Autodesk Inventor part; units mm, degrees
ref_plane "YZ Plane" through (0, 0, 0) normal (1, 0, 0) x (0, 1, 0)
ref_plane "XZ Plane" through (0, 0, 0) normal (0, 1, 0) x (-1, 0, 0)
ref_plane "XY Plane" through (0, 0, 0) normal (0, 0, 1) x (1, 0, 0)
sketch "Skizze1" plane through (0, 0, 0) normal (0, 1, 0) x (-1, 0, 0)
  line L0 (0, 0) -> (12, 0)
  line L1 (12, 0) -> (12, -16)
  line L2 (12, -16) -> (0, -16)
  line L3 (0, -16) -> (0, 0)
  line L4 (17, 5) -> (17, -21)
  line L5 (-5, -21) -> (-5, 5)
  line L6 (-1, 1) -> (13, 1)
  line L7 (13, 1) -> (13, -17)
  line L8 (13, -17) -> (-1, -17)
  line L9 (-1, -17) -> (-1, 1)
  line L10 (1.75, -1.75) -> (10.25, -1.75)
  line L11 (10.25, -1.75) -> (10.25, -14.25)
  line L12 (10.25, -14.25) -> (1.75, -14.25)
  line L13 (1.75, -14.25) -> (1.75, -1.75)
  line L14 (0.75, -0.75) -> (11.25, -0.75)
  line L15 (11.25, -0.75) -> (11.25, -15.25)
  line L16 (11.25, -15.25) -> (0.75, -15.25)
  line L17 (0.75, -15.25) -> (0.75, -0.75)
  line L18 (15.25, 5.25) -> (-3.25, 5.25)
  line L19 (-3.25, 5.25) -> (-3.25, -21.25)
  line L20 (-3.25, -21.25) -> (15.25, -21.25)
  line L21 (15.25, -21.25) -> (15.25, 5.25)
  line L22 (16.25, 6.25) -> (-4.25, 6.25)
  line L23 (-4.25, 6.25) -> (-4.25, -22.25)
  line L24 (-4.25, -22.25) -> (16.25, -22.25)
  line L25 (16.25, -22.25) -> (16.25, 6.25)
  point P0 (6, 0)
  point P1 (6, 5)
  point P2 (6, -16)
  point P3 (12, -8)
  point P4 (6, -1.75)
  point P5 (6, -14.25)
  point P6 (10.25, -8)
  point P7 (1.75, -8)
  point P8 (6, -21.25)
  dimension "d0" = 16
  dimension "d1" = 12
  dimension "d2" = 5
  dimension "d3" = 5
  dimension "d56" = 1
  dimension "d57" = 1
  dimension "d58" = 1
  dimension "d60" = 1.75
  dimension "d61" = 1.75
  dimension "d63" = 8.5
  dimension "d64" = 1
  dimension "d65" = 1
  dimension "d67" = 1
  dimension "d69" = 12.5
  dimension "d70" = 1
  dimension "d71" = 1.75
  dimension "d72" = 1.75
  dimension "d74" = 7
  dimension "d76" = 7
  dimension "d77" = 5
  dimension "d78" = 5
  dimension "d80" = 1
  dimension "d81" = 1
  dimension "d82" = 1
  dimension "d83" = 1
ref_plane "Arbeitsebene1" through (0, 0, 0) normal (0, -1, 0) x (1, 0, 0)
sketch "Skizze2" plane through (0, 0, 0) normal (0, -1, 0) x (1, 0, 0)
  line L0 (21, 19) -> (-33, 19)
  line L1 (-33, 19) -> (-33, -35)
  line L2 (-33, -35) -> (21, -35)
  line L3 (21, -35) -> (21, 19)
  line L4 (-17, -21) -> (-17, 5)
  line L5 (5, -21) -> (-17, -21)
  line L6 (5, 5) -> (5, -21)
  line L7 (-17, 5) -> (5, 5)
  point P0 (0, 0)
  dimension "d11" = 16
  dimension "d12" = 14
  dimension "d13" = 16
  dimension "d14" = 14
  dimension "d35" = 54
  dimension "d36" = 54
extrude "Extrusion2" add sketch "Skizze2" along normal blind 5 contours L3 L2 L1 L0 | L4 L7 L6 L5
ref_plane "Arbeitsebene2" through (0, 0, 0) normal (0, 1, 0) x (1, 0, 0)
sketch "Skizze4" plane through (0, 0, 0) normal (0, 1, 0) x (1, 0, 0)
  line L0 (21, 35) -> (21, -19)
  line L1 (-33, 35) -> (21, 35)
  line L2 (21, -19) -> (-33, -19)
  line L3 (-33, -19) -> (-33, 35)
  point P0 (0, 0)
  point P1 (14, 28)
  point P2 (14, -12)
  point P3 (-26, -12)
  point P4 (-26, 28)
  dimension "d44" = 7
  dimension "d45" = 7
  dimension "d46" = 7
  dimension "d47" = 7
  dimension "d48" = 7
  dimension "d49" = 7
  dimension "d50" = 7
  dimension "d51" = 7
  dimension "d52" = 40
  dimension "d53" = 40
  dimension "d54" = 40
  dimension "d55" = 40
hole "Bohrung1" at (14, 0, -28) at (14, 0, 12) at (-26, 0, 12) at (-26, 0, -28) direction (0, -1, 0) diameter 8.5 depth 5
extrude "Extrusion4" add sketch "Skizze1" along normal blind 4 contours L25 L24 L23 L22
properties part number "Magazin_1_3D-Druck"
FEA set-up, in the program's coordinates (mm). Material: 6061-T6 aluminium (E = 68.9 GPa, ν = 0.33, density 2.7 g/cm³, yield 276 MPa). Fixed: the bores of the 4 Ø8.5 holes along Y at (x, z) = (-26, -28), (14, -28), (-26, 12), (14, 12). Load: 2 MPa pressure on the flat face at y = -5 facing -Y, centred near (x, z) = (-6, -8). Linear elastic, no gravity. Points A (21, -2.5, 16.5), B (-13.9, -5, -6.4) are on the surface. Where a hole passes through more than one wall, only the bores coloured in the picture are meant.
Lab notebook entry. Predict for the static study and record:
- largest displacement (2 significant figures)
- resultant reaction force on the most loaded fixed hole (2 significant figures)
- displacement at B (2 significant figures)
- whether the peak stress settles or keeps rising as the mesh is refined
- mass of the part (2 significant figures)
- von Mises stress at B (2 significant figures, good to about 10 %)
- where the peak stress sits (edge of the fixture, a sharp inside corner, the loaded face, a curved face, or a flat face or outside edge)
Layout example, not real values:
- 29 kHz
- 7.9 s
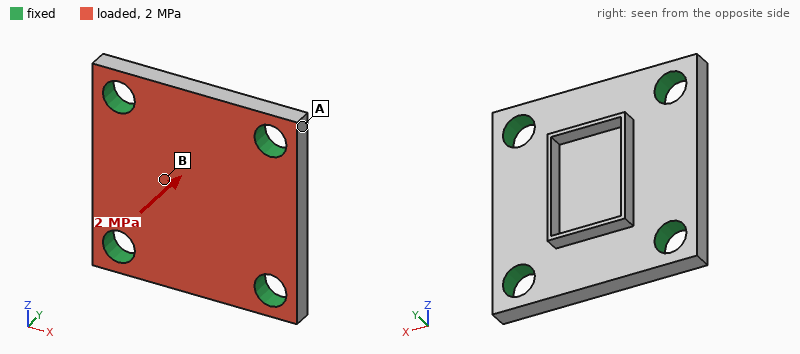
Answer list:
- 27 µm
- 1.3 kN
- 23 µm
- keeps rising
- 37 g
- 22 MPa
- edge of the fixture
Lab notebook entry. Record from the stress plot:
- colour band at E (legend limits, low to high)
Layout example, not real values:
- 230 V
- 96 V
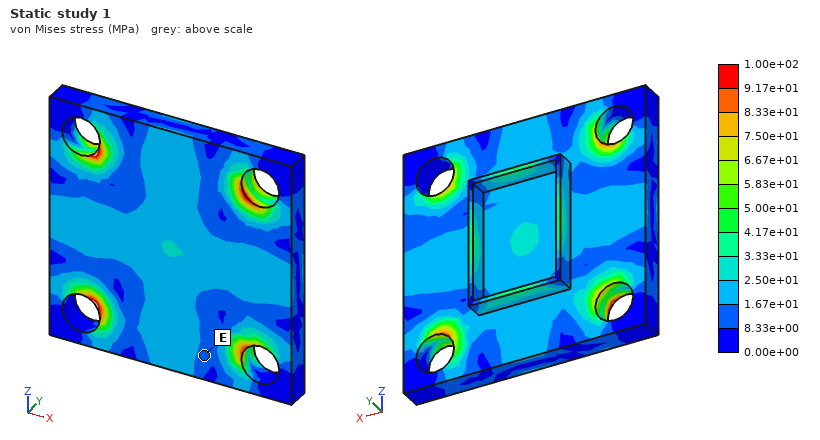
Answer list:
- 8.33e+00 to 1.67e+01 MPa
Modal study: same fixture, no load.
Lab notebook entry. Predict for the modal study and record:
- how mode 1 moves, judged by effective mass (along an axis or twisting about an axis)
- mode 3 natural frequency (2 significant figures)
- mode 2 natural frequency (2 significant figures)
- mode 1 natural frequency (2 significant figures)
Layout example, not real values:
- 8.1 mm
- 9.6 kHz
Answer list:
- along Y
- 21 kHz
- 21 kHz
- 14 kHz
